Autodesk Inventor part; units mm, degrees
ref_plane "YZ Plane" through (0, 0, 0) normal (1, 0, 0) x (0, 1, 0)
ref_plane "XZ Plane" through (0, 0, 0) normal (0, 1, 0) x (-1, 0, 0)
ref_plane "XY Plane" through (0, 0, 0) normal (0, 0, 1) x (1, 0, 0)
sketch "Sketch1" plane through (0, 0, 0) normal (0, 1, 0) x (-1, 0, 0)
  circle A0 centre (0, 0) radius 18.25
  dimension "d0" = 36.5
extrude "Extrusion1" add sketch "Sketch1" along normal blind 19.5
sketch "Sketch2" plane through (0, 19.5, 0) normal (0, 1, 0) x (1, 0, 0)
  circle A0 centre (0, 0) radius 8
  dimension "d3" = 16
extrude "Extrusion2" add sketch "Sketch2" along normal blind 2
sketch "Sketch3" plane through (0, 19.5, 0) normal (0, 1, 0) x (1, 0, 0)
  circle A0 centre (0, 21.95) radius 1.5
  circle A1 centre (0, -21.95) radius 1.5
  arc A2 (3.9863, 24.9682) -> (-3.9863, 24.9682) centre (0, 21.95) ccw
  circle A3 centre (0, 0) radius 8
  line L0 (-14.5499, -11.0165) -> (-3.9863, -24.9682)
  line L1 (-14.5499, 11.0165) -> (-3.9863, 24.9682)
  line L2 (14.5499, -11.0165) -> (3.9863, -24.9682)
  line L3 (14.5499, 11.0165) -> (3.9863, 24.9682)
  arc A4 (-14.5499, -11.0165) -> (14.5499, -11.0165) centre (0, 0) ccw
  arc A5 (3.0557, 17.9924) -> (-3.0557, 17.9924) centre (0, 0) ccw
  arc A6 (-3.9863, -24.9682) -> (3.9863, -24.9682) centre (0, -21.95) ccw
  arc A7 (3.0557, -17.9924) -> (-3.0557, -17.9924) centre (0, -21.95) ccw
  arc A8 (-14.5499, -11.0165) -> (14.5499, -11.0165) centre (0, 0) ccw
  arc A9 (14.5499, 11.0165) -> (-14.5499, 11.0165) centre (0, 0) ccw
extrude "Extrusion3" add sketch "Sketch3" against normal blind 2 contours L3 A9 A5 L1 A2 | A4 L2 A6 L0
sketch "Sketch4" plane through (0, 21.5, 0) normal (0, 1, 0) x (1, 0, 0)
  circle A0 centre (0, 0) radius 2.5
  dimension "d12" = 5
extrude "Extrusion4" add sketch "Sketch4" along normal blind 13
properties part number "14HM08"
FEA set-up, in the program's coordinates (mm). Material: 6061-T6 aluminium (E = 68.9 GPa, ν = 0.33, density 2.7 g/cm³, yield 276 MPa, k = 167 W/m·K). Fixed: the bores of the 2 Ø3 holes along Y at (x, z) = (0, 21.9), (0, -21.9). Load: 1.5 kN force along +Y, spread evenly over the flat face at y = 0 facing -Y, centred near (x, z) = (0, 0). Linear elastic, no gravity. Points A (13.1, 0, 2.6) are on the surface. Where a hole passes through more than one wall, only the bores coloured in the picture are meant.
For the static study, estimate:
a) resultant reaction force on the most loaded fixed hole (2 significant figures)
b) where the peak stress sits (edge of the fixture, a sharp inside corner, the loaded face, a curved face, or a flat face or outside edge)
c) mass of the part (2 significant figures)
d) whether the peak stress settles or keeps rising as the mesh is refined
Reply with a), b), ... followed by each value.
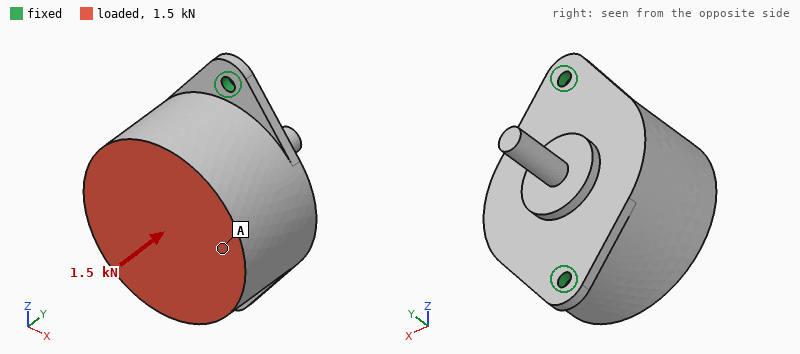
a) 850 N
b) edge of the fixture
c) 58 g
d) keeps rising
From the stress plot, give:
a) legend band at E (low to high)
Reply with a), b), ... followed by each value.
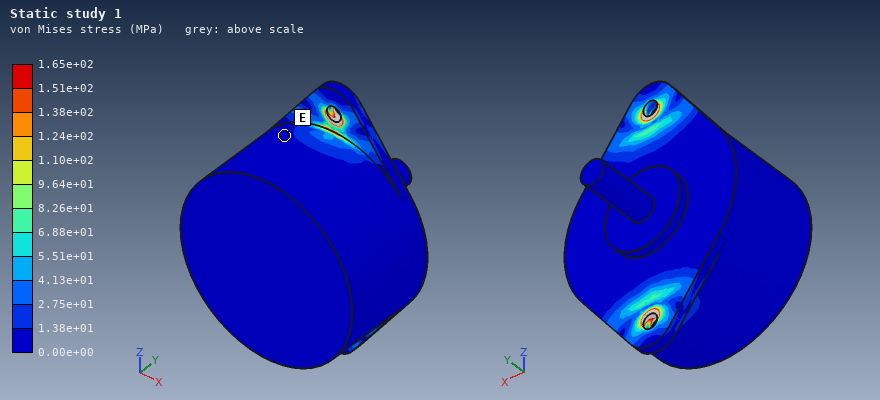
a) 0.00e+00 to 1.38e+01 MPa
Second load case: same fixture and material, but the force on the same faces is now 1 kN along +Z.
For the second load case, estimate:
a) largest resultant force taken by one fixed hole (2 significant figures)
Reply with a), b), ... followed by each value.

a) 690 N
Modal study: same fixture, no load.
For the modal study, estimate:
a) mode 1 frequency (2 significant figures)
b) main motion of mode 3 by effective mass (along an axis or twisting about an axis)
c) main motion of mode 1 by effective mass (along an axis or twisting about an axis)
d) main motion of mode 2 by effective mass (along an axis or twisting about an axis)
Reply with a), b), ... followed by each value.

a) 1200 Hz
b) along Z
c) along X
d) along Y
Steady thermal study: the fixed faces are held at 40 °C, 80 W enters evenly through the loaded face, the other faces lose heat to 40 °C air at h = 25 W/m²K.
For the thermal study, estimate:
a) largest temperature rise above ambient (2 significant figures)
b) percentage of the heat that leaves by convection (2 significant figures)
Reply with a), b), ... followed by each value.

a) 64 K
b) 6.7 %
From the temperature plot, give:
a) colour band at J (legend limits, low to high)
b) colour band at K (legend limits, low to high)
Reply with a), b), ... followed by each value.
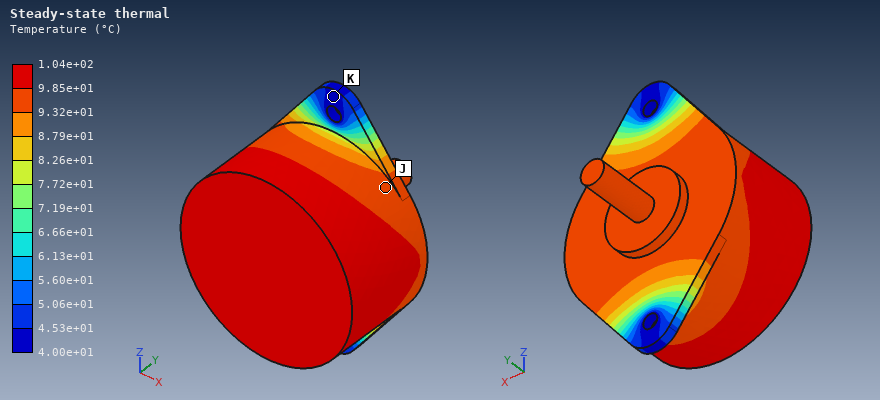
a) 9.32e+01 to 9.85e+01 °C
b) 4.00e+01 to 4.53e+01 °C
